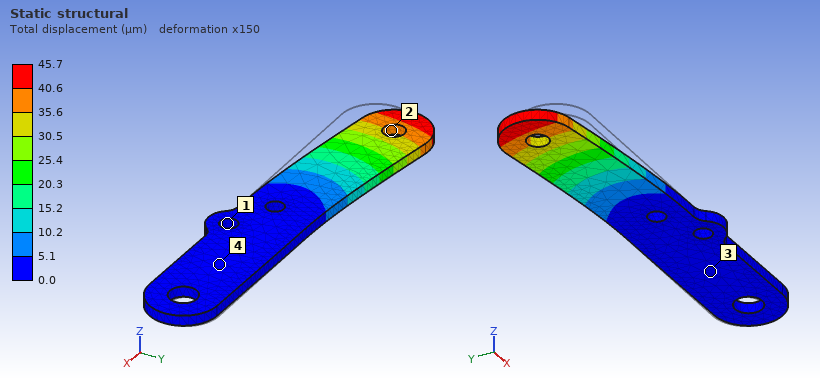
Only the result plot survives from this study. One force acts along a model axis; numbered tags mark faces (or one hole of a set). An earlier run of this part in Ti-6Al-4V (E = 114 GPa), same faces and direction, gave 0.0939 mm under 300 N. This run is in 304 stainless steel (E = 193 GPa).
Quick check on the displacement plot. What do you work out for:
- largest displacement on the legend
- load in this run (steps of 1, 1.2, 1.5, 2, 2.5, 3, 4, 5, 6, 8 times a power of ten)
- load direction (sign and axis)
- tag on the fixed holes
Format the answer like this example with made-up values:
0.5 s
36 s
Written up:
45.7 µm
250 N
+Y
1
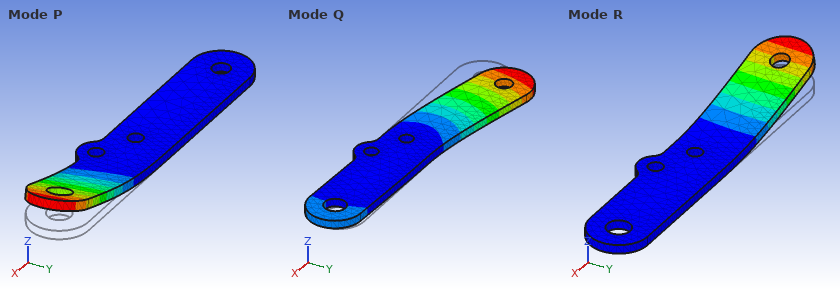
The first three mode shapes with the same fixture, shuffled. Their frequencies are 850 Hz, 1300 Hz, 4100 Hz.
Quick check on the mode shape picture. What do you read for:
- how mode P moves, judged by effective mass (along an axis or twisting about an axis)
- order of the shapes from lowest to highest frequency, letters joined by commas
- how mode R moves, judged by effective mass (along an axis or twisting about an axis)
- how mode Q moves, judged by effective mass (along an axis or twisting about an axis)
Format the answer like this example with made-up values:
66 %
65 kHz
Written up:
along Z
R, P, Q
along Z
along Y
